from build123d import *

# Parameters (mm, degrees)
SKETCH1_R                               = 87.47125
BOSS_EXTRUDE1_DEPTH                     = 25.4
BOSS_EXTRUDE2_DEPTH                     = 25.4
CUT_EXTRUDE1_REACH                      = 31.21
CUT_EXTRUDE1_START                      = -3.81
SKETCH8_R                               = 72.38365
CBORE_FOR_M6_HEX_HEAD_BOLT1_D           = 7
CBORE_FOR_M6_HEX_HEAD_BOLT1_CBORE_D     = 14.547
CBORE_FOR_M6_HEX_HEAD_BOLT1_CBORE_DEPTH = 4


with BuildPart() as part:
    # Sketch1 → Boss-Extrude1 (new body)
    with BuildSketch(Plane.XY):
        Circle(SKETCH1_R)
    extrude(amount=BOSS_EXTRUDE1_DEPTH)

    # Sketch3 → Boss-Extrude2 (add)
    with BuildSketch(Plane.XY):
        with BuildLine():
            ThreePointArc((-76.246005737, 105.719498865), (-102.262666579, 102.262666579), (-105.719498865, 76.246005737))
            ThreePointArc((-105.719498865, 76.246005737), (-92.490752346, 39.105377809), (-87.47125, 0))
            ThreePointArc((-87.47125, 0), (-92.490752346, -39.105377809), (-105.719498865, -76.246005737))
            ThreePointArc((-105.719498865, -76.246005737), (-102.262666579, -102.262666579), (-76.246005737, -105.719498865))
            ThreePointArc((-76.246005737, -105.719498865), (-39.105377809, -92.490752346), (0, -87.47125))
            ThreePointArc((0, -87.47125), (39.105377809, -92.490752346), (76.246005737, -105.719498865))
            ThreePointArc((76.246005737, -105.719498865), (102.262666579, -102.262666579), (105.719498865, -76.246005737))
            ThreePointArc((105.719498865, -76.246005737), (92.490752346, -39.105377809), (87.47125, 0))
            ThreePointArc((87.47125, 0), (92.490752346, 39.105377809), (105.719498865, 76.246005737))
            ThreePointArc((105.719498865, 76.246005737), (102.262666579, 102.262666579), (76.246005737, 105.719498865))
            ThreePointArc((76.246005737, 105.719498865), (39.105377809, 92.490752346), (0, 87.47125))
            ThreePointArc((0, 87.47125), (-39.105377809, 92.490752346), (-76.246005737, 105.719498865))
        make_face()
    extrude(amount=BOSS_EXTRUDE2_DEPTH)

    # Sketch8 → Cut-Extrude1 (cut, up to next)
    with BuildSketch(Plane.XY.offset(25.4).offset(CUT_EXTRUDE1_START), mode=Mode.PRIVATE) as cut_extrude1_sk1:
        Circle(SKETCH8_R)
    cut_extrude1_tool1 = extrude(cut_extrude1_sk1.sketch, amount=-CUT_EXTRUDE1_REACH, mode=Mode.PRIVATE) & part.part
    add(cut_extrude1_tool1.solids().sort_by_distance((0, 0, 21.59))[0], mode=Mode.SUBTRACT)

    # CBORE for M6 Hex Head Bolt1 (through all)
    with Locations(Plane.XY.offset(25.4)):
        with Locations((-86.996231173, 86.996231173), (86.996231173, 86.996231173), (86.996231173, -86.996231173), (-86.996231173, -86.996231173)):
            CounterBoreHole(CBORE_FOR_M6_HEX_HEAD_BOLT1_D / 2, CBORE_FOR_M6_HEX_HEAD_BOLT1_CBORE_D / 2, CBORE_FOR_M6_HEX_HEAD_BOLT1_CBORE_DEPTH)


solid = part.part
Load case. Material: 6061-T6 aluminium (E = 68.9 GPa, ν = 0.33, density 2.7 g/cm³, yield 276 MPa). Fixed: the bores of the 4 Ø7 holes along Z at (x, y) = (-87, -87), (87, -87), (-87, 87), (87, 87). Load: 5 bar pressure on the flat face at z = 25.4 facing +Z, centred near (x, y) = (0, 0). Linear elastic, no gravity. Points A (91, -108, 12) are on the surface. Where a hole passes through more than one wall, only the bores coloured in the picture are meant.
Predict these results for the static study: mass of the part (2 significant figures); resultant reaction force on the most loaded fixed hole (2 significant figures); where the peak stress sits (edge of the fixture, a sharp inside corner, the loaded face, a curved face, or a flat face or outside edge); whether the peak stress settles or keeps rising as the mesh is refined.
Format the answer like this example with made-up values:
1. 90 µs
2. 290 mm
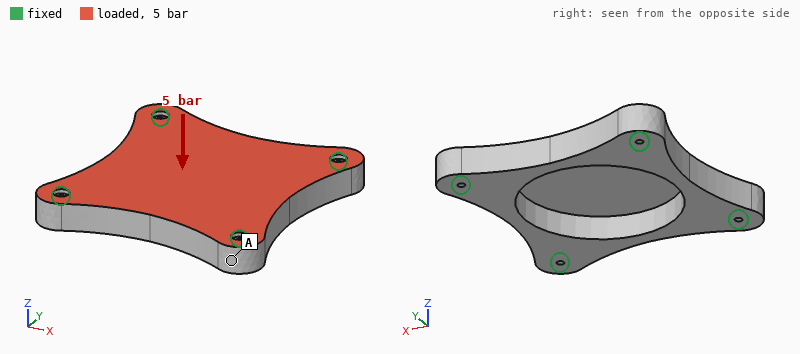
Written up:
1. 1.6 kg
2. 6.0 kN
3. edge of the fixture
4. keeps rising
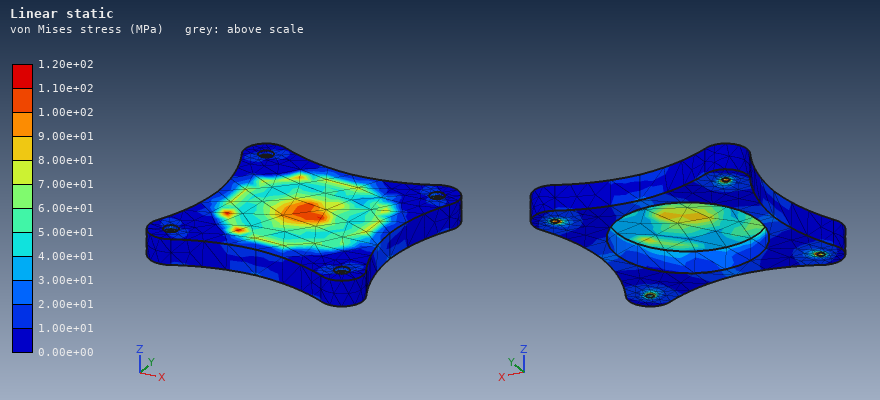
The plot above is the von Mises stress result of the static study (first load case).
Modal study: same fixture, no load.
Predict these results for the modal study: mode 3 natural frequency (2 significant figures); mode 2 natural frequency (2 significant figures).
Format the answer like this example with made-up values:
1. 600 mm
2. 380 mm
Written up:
1. 3300 Hz
2. 3300 Hz
